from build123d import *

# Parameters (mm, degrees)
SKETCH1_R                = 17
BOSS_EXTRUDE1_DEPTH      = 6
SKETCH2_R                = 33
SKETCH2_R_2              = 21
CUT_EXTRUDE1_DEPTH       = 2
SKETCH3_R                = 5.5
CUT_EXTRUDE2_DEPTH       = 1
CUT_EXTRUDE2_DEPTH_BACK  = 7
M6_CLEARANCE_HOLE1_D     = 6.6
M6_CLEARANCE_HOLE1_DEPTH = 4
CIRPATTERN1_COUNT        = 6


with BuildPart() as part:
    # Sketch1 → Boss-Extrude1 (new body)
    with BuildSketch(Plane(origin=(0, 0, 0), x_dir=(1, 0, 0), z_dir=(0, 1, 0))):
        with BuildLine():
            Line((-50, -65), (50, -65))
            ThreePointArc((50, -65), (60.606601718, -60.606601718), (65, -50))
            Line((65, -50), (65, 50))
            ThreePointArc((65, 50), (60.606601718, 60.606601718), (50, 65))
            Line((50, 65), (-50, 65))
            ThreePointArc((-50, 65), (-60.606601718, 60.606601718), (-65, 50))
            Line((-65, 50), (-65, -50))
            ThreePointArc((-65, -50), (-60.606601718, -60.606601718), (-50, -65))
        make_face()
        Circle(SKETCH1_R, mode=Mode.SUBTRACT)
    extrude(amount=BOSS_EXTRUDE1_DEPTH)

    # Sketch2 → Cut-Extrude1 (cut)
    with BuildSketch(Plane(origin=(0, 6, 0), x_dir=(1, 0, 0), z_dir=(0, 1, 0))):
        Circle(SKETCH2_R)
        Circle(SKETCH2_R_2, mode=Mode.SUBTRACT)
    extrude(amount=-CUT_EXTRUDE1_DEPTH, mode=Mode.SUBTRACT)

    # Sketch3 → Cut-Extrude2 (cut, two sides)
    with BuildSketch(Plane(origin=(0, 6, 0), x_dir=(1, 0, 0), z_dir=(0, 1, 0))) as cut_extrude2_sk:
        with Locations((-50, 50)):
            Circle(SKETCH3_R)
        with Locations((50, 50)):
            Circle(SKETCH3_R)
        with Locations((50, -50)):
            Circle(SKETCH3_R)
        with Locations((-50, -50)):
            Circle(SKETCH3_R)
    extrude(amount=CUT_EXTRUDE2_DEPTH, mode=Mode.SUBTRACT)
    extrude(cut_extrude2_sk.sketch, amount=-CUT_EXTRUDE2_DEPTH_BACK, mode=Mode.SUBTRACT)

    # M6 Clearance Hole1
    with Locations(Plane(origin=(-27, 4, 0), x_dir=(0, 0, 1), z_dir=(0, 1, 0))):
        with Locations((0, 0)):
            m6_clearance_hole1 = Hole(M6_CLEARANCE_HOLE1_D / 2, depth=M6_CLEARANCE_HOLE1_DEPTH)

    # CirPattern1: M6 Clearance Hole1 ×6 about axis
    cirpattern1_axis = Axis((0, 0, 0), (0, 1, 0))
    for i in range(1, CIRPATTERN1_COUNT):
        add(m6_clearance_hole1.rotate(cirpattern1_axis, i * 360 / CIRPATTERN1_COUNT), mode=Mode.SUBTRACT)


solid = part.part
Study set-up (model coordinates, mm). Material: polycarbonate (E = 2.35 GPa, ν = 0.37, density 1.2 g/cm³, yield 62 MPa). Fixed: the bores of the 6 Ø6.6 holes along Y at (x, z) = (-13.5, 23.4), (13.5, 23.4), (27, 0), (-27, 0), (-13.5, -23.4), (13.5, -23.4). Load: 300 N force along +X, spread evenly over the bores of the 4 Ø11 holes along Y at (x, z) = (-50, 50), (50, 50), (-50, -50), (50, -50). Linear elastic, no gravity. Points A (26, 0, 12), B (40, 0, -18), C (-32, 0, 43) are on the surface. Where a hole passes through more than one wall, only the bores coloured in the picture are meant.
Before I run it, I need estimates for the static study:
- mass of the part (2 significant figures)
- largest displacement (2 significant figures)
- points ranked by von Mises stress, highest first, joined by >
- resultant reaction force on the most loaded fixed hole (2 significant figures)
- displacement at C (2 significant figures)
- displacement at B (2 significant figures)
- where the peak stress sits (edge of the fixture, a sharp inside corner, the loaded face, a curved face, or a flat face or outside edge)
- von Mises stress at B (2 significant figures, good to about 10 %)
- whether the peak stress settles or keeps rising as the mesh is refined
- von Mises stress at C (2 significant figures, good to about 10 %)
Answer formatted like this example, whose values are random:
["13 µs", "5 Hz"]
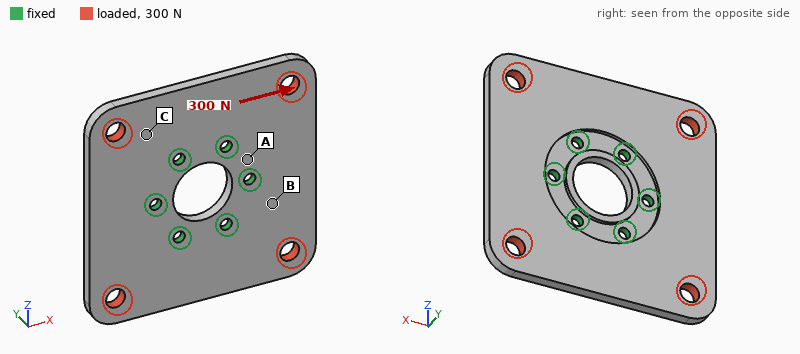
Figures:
["110 g", "26 µm", "C > B > A", "64 N", "11 µm", "7.0 µm", "edge of the fixture", "0.25 MPa", "keeps rising", "0.37 MPa"]
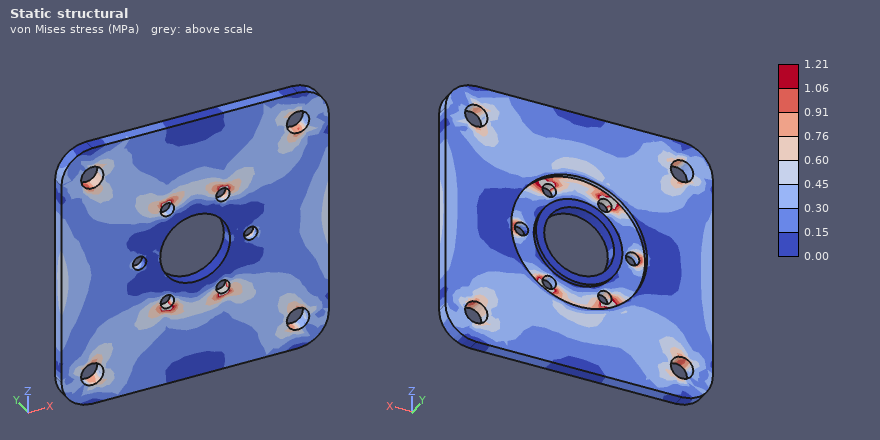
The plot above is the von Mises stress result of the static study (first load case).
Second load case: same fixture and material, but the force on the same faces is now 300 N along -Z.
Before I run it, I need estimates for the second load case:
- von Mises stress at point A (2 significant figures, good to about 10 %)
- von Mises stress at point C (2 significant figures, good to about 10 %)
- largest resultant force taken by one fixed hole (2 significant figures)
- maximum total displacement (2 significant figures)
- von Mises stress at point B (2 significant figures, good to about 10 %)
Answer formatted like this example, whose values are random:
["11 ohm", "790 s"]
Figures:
["0.45 MPa", "0.41 MPa", "77 N", "26 µm", "0.35 MPa"]
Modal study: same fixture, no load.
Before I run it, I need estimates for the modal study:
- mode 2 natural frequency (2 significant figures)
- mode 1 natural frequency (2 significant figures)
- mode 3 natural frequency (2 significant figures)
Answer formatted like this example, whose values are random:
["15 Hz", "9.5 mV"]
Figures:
["450 Hz", "450 Hz", "460 Hz"]
